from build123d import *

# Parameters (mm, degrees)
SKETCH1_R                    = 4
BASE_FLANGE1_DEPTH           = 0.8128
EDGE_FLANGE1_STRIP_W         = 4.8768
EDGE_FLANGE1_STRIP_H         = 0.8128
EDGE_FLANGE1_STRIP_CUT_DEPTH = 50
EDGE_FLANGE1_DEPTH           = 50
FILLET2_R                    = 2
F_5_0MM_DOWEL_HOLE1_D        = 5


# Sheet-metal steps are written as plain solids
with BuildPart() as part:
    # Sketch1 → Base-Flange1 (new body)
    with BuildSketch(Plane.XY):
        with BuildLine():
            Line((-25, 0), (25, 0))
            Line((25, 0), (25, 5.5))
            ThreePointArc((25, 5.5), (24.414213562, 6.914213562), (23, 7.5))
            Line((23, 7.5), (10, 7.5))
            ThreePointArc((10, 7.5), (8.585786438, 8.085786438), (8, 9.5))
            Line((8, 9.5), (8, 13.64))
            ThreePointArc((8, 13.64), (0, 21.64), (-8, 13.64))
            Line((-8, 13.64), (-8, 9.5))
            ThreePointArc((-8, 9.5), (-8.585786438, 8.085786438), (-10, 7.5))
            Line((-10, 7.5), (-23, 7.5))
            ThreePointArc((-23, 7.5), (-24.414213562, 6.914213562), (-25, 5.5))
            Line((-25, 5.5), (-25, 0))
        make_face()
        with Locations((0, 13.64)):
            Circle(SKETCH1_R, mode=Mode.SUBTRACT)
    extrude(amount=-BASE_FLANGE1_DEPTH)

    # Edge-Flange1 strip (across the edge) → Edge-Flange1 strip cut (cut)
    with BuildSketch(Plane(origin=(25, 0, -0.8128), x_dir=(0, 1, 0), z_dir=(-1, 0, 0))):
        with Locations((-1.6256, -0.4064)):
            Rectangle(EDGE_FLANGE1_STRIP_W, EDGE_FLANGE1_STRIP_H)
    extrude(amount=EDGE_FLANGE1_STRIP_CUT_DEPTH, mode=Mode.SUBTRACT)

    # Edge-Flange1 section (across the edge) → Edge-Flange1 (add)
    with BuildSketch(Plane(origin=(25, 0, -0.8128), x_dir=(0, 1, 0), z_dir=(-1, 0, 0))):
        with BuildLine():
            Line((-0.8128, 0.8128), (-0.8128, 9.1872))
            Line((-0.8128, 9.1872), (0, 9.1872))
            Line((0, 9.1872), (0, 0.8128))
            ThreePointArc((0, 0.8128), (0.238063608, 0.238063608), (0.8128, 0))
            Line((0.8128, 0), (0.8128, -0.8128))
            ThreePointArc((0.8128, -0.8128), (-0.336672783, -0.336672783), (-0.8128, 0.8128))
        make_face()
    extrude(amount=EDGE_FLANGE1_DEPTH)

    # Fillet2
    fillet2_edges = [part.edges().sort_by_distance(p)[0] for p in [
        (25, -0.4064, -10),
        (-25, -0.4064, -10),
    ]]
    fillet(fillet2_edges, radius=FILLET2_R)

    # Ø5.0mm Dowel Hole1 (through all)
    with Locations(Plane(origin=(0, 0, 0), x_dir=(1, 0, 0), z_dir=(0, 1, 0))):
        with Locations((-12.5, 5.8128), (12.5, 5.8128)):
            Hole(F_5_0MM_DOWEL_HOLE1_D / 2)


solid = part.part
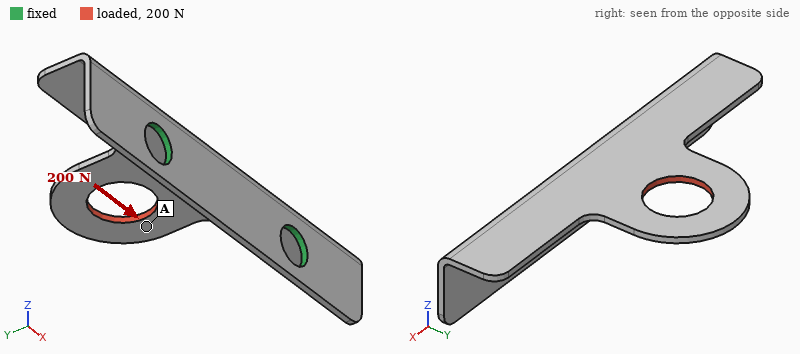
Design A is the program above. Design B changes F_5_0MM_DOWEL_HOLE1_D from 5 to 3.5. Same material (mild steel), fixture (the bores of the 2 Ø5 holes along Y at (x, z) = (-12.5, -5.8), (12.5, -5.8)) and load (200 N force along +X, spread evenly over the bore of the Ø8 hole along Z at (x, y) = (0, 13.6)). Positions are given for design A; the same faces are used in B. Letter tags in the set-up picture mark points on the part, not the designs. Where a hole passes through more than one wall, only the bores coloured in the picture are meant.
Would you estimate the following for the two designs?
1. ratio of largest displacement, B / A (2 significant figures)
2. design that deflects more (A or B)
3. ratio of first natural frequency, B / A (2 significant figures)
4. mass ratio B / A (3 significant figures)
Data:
1.6
B
0.96
1.02
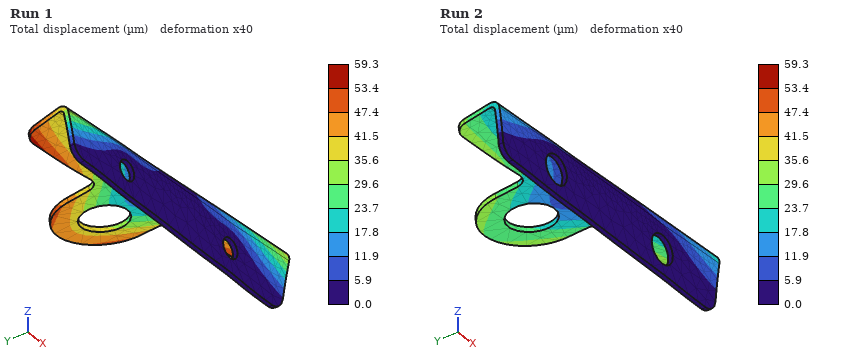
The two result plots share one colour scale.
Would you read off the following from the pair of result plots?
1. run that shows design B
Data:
Run 1
